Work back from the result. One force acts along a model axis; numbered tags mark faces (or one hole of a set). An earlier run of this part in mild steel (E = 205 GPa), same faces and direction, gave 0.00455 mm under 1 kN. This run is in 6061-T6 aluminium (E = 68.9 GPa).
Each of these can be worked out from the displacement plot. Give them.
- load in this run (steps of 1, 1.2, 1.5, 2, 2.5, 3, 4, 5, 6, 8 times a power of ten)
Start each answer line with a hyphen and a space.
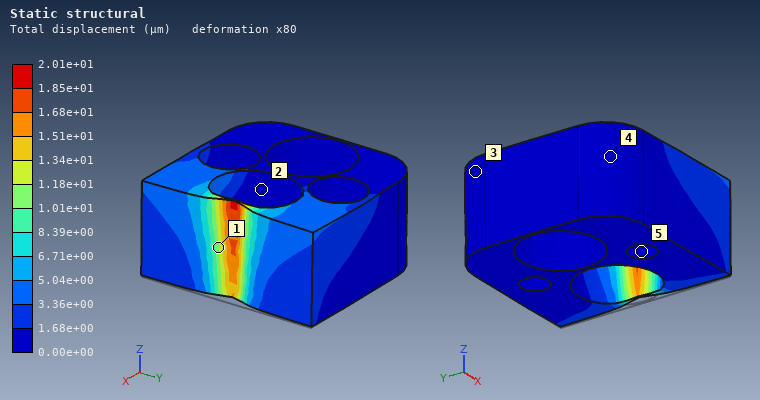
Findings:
- 1.5 kN
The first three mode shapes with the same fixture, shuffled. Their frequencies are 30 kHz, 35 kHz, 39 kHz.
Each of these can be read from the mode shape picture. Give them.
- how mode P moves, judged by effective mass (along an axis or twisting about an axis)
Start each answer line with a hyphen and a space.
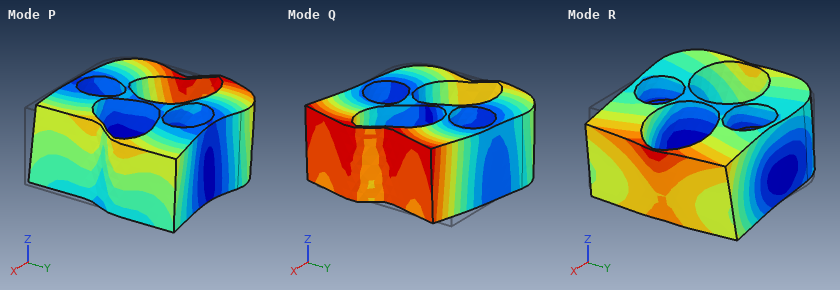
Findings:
- along Y
